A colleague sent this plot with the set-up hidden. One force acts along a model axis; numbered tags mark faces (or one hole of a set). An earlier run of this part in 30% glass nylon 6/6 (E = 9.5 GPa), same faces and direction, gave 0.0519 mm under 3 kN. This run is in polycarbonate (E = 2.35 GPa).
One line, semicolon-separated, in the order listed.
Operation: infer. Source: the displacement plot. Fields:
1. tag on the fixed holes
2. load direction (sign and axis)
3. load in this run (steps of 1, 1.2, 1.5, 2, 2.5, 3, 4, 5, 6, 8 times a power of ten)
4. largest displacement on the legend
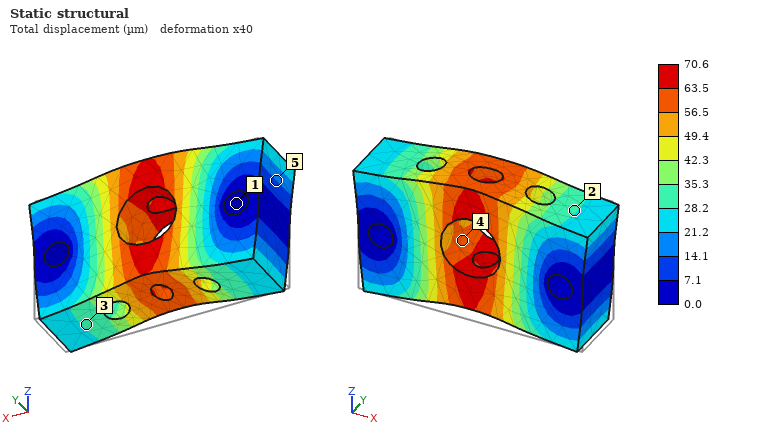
1; +Z; 1 kN; 70.6 µm
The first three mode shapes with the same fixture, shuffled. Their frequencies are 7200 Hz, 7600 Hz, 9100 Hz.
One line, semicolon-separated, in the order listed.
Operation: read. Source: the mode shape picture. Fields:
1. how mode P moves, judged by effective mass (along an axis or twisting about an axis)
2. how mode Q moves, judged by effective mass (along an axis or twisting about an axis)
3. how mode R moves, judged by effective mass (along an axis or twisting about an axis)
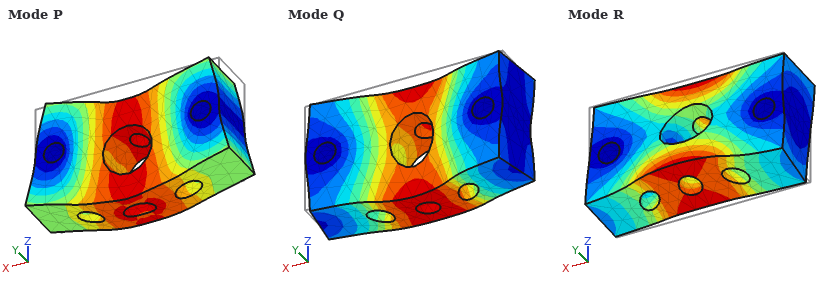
along Z; along Y; twisting about X
